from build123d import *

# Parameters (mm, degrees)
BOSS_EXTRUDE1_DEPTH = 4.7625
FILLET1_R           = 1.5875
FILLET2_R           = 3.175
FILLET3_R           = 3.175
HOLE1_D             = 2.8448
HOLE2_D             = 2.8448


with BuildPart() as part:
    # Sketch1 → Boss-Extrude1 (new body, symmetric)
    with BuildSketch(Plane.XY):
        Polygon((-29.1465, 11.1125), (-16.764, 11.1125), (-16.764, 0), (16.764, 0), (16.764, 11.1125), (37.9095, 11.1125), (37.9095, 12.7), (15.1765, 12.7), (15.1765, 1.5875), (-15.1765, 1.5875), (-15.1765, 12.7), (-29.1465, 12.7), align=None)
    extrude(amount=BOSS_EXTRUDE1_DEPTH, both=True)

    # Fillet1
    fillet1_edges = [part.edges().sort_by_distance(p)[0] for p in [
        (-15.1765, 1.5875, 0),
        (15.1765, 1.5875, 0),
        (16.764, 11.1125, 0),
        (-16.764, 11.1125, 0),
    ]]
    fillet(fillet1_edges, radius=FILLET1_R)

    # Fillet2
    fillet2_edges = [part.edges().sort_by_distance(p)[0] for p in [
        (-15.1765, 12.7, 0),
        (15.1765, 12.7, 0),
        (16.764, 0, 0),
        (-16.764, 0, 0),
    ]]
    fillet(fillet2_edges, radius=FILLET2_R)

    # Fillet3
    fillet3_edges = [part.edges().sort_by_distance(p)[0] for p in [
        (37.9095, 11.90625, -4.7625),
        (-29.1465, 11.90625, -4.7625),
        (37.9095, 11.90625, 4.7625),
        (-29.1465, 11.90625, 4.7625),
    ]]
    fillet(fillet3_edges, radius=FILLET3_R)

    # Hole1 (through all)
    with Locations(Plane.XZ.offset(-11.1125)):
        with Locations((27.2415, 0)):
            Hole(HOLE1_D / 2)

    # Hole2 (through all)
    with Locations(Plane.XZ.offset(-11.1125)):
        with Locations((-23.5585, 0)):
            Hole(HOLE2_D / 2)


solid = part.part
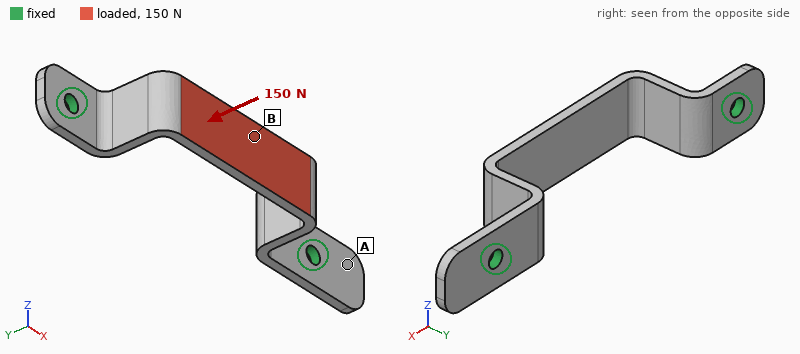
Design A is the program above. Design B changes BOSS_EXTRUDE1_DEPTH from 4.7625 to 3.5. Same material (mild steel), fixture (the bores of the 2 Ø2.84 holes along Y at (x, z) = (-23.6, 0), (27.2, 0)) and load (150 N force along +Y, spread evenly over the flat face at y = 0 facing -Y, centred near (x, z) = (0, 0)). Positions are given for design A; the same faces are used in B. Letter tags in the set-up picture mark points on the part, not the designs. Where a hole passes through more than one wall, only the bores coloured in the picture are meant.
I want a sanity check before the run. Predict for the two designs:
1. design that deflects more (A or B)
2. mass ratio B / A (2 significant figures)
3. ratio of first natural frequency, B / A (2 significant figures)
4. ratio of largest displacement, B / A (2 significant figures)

B
0.73
0.98
1.3
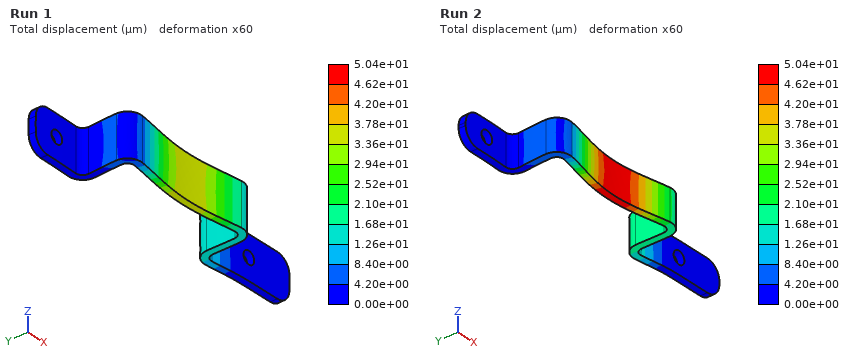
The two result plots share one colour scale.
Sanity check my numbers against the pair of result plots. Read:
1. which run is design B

Run 2
